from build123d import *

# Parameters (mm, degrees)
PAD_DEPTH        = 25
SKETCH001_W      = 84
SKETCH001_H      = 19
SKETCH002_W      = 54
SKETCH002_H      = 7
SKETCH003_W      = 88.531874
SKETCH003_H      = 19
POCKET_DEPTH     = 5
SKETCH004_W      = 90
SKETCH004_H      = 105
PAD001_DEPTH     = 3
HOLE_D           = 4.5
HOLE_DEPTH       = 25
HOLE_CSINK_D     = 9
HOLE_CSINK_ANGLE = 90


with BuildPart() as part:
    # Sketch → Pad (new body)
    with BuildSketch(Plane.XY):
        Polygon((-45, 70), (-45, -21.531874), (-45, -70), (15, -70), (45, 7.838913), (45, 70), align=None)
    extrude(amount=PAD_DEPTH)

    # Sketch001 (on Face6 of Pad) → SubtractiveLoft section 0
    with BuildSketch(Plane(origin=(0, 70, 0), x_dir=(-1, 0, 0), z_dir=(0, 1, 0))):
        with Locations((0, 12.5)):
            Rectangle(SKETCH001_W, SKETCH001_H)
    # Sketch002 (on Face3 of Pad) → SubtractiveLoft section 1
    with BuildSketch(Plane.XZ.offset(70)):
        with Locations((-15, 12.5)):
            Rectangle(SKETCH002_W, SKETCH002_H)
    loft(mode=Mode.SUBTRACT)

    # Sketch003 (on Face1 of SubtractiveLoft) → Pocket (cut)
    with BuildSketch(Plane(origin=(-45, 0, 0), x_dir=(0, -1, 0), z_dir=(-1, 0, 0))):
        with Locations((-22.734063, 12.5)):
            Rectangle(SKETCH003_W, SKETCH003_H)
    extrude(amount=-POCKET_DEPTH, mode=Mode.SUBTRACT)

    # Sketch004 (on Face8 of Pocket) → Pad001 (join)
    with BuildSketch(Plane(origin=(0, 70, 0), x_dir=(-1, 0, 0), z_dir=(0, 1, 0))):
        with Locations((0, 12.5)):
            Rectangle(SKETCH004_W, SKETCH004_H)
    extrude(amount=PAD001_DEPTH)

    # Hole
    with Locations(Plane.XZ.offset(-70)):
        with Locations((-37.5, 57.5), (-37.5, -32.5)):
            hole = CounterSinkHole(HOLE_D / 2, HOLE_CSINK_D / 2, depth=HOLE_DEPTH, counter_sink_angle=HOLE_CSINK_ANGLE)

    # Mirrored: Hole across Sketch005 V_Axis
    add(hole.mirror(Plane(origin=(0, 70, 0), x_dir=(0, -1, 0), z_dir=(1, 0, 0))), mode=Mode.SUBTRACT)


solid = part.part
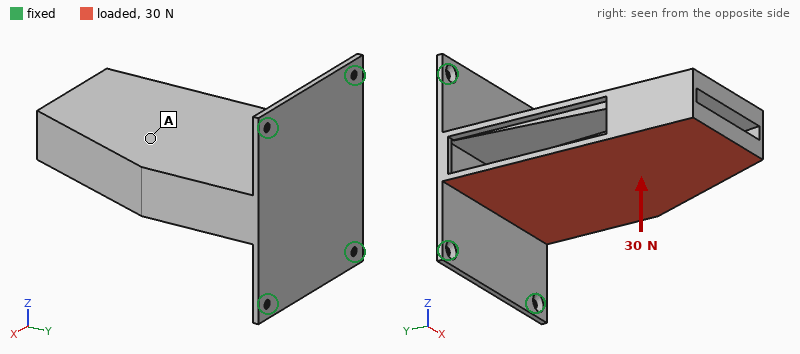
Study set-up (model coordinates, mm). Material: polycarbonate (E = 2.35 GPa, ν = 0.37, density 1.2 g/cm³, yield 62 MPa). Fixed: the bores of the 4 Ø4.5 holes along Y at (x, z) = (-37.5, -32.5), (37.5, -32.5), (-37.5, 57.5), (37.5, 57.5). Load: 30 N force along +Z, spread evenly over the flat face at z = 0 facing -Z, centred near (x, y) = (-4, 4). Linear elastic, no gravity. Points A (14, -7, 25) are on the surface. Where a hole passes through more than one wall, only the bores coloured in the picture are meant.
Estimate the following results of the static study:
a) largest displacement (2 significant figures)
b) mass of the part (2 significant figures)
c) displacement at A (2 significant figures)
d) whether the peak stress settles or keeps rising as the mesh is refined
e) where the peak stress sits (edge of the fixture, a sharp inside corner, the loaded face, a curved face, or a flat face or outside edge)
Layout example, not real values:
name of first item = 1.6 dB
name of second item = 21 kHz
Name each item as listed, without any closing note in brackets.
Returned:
largest displacement = 1.9 mm
mass of the part = 210 g
displacement at A = 1.0 mm
whether the peak stress settles or keeps rising as the mesh is refined = keeps rising
where the peak stress sits = edge of the fixture
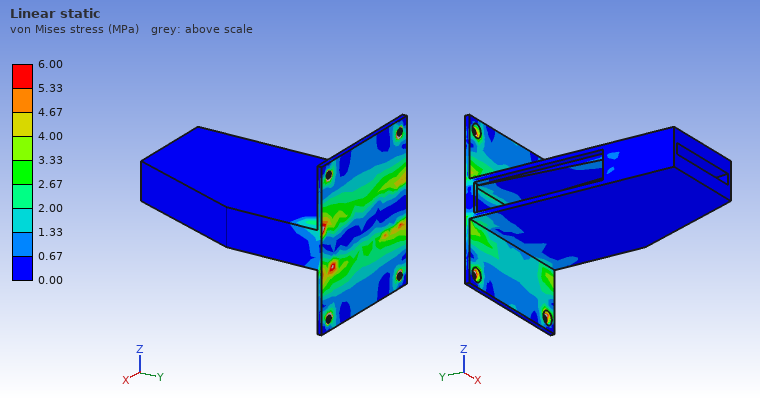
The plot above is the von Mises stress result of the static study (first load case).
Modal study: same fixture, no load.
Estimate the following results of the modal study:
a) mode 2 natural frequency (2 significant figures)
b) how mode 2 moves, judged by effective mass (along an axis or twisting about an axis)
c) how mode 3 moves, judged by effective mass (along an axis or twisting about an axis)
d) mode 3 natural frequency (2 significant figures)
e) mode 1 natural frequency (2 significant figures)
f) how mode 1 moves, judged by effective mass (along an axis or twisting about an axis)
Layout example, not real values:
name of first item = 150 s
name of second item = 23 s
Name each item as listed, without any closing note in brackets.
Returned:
mode 2 natural frequency = 56 Hz
how mode 2 moves, judged by effective mass = along X
how mode 3 moves, judged by effective mass = along Y
mode 3 natural frequency = 130 Hz
mode 1 natural frequency = 53 Hz
how mode 1 moves, judged by effective mass = along Z
